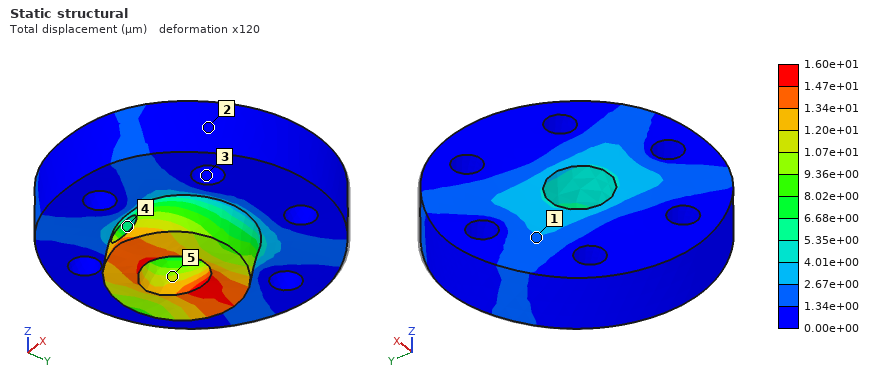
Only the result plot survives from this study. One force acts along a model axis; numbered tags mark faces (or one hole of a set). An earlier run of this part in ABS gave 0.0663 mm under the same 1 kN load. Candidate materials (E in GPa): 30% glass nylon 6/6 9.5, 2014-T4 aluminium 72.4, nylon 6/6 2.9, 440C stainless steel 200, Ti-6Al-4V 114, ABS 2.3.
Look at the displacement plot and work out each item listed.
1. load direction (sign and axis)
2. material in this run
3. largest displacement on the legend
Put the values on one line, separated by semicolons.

-Y; 30% glass nylon 6/6; 1.60e+01 µm
